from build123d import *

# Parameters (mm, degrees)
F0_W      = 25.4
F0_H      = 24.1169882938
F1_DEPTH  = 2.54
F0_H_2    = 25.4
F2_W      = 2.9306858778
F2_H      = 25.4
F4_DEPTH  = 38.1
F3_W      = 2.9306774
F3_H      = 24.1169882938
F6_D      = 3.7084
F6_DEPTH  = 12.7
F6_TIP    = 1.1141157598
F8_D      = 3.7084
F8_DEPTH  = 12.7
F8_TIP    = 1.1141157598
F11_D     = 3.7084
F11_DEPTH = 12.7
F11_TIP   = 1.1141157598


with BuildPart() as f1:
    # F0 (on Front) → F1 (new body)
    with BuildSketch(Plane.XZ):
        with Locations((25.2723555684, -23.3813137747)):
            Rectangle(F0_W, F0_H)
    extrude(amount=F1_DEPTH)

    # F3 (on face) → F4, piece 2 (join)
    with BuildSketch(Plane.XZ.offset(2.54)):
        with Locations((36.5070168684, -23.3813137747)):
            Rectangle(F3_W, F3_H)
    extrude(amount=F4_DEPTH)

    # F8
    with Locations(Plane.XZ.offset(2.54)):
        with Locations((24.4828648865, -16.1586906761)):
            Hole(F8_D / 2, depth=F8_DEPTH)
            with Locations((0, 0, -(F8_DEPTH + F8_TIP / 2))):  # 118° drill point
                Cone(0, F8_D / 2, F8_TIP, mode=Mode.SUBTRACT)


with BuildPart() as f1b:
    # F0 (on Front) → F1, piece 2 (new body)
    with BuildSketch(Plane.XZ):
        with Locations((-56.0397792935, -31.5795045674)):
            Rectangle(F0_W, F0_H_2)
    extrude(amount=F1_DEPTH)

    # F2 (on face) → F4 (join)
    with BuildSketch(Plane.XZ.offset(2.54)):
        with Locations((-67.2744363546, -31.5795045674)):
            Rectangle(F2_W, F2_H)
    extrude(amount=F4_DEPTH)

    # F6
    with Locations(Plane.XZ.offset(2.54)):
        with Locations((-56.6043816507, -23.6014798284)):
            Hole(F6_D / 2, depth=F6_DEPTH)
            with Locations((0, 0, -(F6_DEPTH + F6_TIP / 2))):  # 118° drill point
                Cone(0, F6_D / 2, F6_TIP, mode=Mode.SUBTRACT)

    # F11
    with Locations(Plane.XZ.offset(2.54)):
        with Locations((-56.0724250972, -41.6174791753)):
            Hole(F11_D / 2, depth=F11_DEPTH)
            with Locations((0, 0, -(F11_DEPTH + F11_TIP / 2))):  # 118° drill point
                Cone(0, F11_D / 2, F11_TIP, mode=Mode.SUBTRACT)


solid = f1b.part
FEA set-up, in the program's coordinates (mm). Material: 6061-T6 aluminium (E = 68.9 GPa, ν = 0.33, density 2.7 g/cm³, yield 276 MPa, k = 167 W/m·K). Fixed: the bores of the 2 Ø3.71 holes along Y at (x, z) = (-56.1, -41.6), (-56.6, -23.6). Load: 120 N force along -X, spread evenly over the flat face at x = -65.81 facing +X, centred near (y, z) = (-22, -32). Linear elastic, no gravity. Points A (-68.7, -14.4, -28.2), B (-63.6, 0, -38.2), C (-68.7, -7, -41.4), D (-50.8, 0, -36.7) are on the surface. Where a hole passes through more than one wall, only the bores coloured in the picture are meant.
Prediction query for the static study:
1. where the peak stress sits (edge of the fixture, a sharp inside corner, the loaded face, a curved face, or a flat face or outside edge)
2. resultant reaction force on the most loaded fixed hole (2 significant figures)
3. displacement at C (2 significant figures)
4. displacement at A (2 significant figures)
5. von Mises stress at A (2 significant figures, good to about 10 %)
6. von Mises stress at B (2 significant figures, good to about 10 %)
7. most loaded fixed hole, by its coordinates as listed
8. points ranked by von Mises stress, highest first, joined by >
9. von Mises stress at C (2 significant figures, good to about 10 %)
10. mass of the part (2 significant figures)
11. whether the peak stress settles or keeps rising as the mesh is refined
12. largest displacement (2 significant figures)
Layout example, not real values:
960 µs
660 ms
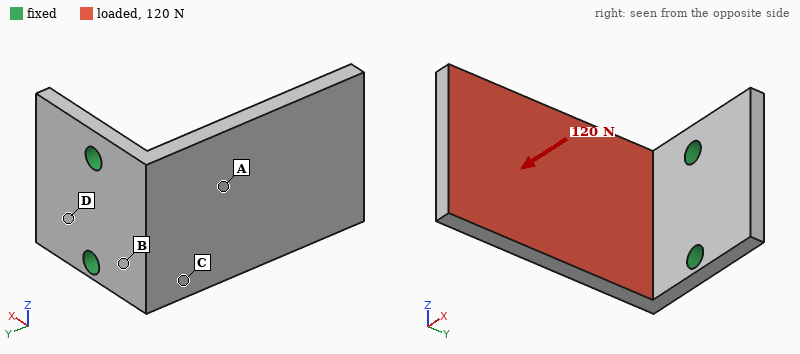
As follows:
edge of the fixture
71 N
0.094 mm
0.18 mm
27 MPa
75 MPa
(-56.6, -23.6)
B > C > A > D
47 MPa
12 g
keeps rising
0.61 mm
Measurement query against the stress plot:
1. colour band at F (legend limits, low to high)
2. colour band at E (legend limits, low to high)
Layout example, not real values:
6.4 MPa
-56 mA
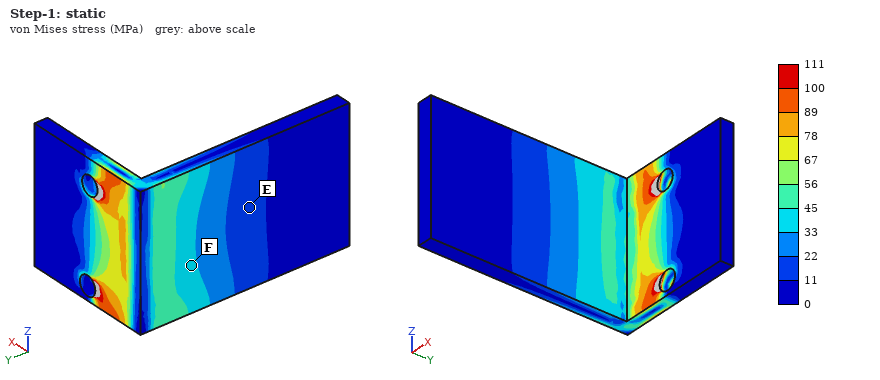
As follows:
33 to 45 MPa
11 to 22 MPa
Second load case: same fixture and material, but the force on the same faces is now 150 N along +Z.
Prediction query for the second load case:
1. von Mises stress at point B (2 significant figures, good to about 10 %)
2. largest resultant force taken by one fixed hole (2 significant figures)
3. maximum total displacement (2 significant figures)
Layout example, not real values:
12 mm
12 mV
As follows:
33 MPa
190 N
0.12 mm
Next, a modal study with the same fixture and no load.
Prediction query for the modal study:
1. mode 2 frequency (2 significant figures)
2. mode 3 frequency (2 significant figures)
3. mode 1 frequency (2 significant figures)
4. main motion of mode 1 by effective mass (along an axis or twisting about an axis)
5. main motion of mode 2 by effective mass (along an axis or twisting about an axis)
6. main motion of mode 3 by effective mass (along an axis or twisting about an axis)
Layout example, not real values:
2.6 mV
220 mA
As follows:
2500 Hz
5000 Hz
990 Hz
along X
along Z
twisting about Y
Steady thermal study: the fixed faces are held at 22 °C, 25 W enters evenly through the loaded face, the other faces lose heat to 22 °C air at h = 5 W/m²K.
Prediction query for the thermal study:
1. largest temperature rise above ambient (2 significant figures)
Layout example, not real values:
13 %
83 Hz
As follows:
63 K
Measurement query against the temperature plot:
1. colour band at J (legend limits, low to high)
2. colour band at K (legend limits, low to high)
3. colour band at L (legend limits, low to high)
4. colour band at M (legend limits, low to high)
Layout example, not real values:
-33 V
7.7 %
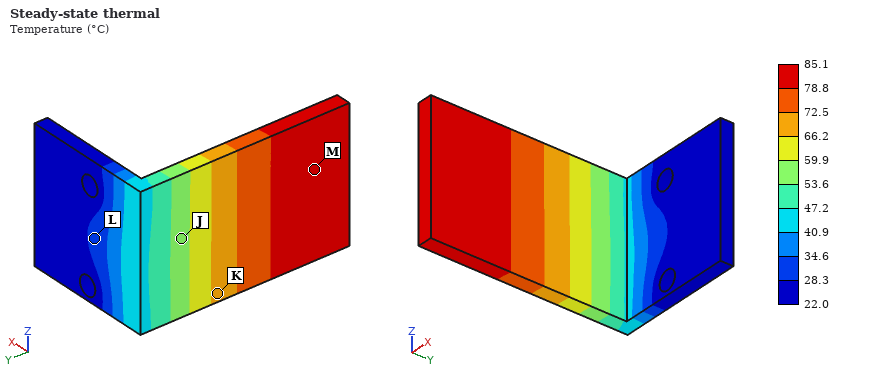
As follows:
53.6 to 59.9 °C
66.2 to 72.5 °C
28.3 to 34.6 °C
78.8 to 85.1 °C
